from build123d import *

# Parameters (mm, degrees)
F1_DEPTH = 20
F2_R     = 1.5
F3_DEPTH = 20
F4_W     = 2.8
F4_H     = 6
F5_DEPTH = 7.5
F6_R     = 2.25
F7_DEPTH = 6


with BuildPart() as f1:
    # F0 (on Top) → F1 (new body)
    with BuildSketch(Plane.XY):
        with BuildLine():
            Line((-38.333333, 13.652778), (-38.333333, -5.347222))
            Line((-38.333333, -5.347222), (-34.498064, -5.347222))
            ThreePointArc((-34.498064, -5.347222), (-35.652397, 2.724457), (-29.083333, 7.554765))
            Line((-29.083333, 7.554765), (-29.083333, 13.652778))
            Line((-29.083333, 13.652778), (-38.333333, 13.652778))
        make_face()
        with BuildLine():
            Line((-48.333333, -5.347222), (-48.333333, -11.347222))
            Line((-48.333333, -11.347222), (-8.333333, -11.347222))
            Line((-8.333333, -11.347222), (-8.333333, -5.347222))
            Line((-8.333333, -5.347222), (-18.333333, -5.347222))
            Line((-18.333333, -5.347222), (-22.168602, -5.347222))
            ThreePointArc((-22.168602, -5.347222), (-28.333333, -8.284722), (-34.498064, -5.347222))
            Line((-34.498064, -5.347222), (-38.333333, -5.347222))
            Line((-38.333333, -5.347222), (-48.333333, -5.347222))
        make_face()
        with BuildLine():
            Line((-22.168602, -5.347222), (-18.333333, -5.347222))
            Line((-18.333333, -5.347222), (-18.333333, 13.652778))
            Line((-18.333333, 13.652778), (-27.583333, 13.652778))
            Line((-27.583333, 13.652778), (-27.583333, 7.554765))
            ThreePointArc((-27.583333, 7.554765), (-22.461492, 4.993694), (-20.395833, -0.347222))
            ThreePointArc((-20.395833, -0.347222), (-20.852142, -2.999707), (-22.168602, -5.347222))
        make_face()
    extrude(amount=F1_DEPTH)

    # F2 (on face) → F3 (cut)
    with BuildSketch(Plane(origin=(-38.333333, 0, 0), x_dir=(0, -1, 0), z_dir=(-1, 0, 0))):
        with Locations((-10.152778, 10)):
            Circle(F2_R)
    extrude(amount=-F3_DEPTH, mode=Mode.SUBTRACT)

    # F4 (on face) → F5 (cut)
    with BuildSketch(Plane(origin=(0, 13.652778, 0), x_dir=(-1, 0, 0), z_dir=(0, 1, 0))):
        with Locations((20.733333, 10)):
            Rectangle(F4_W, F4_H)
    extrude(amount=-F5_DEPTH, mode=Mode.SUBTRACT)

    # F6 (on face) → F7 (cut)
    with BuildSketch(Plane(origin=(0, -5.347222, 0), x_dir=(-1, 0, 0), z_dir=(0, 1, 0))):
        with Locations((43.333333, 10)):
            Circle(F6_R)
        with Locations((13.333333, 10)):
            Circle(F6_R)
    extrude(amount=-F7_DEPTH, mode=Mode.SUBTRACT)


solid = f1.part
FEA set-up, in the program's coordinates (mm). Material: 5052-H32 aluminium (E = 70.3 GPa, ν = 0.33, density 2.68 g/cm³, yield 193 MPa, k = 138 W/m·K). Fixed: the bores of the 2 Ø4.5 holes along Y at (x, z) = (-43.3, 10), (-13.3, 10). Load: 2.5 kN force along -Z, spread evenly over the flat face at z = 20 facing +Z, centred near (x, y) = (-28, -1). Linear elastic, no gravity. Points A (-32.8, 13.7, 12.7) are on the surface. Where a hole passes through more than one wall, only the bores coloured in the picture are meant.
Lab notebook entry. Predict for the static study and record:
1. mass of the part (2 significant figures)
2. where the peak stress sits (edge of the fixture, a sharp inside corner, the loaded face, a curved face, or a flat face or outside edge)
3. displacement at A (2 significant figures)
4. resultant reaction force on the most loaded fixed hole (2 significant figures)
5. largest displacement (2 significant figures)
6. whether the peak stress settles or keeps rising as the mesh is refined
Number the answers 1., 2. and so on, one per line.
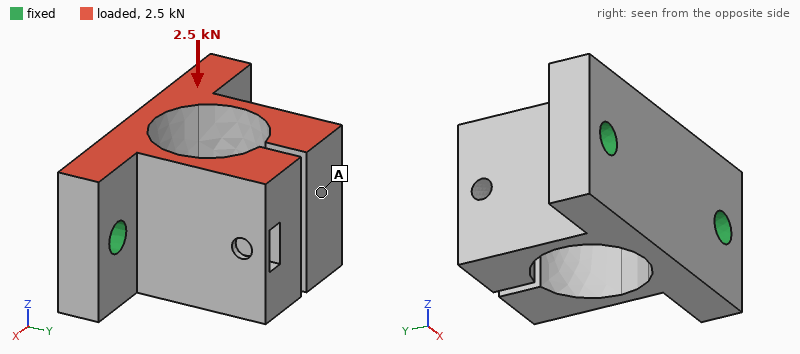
1. 21 g
2. edge of the fixture
3. 58 µm
4. 1.3 kN
5. 70 µm
6. keeps rising
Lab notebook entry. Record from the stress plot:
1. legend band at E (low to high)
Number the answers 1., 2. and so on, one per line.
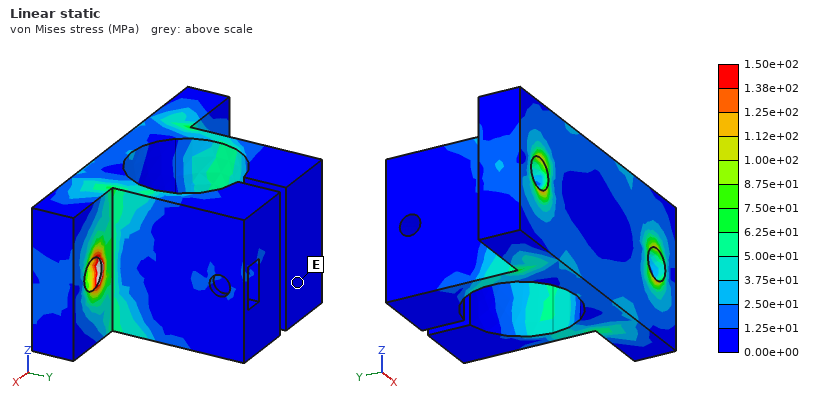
1. 0.00e+00 to 1.25e+01 MPa
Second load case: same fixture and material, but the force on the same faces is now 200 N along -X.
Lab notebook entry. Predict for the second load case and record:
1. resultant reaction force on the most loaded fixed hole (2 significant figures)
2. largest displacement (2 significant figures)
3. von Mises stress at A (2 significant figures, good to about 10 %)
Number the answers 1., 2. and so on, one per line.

1. 120 N
2. 46 µm
3. 2.3 MPa
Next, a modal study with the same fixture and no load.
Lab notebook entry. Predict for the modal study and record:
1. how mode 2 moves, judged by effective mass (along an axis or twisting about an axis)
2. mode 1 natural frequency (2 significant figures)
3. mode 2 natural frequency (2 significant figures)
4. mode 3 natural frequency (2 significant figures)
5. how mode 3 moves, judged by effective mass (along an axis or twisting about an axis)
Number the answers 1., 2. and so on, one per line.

1. along X
2. 2800 Hz
3. 3000 Hz
4. 7600 Hz
5. along Z
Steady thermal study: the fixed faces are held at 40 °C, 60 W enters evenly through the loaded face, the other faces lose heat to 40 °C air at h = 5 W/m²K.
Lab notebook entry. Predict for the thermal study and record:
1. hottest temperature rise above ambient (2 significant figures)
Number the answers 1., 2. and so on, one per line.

1. 44 K
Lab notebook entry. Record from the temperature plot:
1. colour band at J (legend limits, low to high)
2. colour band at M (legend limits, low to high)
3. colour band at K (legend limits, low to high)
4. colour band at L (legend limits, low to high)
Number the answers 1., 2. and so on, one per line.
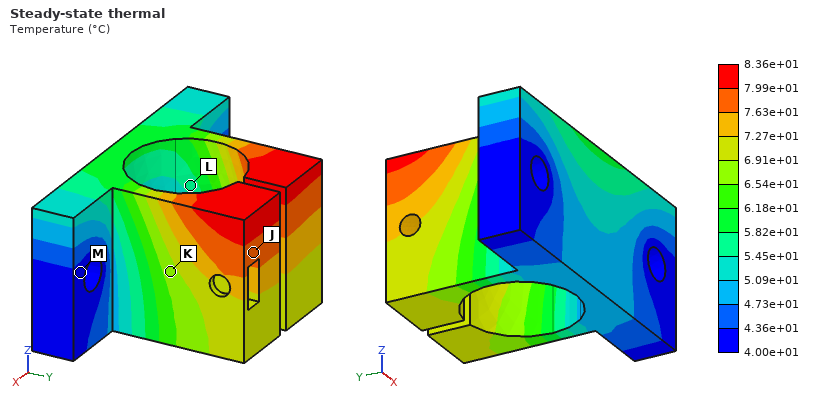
1. 7.63e+01 to 7.99e+01 °C
2. 4.00e+01 to 4.36e+01 °C
3. 6.54e+01 to 6.91e+01 °C
4. 5.45e+01 to 5.82e+01 °C
